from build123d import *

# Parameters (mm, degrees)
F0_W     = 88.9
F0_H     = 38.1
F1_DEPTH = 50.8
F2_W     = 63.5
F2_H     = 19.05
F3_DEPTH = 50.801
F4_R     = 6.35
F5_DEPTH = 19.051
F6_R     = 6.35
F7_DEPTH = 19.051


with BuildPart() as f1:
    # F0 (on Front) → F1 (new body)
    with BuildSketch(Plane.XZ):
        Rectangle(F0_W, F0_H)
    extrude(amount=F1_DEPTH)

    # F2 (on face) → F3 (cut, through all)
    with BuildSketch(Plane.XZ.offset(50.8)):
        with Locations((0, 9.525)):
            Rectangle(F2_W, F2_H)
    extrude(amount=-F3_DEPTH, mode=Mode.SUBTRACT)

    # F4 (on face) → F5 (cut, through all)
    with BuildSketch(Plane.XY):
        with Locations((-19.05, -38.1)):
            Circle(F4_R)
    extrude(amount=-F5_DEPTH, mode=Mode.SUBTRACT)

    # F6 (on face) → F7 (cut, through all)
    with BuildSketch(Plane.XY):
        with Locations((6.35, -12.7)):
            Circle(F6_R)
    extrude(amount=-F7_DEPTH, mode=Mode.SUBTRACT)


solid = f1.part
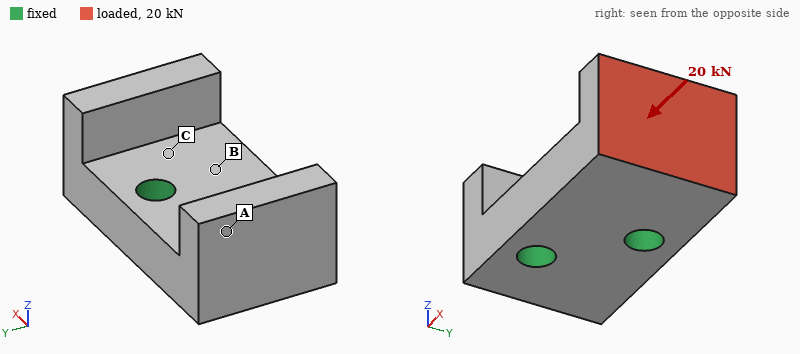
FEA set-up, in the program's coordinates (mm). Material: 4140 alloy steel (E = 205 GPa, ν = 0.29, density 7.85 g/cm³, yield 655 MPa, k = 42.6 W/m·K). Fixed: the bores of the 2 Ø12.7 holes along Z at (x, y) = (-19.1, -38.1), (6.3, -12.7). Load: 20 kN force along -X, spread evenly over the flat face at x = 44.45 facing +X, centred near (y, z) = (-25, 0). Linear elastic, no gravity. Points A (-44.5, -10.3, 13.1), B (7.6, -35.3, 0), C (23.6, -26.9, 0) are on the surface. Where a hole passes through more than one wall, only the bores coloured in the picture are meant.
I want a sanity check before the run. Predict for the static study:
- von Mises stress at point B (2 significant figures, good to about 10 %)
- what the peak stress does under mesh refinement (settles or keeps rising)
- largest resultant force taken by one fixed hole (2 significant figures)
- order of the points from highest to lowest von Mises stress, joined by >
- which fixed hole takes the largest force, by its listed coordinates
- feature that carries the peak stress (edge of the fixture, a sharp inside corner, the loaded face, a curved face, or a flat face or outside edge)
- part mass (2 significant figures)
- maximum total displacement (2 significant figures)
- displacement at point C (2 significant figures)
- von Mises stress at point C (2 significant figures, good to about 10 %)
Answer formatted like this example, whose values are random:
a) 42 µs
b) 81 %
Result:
a) 53 MPa
b) keeps rising
c) 12 kN
d) C > B > A
e) (6.3, -12.7)
f) edge of the fixture
g) 830 g
h) 55 µm
i) 10 µm
j) 77 MPa
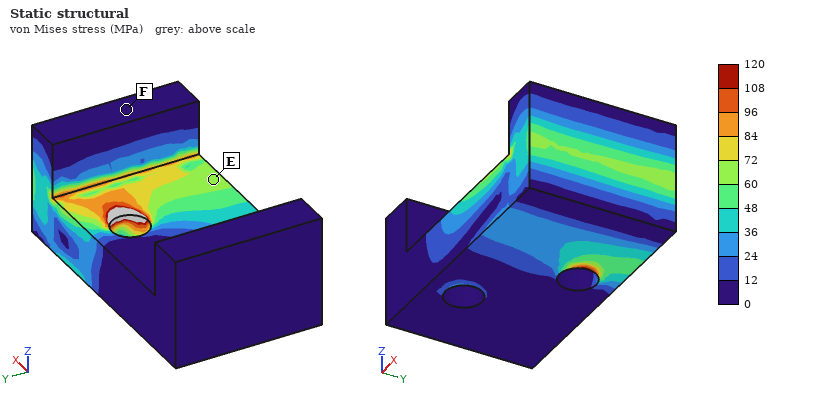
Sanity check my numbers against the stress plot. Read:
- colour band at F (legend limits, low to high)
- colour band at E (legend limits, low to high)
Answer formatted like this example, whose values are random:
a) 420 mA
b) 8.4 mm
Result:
a) 0 to 12 MPa
b) 60 to 72 MPa
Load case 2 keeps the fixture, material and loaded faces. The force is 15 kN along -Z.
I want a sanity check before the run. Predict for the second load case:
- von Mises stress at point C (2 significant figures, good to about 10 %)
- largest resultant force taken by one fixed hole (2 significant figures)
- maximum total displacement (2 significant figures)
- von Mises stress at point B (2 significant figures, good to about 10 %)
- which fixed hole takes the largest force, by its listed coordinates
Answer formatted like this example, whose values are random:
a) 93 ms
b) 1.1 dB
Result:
a) 94 MPa
b) 17 kN
c) 0.10 mm
d) 90 MPa
e) (6.3, -12.7)
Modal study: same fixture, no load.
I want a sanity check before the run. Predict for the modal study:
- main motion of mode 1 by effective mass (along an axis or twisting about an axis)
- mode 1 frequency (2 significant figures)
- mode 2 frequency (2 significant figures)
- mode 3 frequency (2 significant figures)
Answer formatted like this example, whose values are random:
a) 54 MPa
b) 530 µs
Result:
a) along Z
b) 5500 Hz
c) 7900 Hz
d) 8100 Hz
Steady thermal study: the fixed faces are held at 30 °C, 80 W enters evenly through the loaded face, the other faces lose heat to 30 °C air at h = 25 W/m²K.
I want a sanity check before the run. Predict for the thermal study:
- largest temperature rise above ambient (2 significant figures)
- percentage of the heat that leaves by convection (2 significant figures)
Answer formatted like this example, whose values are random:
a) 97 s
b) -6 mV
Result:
a) 81 K
b) 10 %
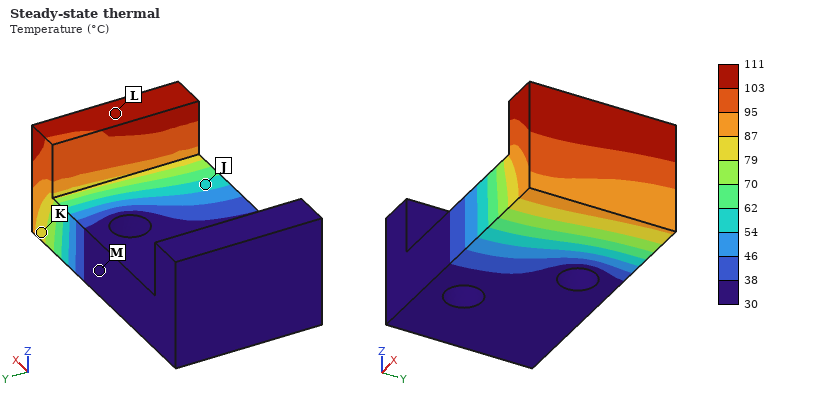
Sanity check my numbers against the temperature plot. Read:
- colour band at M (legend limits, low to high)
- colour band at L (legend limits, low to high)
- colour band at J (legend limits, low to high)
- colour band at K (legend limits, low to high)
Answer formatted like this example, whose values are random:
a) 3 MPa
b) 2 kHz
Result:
a) 30 to 38 °C
b) 103 to 111 °C
c) 54 to 62 °C
d) 79 to 87 °C
